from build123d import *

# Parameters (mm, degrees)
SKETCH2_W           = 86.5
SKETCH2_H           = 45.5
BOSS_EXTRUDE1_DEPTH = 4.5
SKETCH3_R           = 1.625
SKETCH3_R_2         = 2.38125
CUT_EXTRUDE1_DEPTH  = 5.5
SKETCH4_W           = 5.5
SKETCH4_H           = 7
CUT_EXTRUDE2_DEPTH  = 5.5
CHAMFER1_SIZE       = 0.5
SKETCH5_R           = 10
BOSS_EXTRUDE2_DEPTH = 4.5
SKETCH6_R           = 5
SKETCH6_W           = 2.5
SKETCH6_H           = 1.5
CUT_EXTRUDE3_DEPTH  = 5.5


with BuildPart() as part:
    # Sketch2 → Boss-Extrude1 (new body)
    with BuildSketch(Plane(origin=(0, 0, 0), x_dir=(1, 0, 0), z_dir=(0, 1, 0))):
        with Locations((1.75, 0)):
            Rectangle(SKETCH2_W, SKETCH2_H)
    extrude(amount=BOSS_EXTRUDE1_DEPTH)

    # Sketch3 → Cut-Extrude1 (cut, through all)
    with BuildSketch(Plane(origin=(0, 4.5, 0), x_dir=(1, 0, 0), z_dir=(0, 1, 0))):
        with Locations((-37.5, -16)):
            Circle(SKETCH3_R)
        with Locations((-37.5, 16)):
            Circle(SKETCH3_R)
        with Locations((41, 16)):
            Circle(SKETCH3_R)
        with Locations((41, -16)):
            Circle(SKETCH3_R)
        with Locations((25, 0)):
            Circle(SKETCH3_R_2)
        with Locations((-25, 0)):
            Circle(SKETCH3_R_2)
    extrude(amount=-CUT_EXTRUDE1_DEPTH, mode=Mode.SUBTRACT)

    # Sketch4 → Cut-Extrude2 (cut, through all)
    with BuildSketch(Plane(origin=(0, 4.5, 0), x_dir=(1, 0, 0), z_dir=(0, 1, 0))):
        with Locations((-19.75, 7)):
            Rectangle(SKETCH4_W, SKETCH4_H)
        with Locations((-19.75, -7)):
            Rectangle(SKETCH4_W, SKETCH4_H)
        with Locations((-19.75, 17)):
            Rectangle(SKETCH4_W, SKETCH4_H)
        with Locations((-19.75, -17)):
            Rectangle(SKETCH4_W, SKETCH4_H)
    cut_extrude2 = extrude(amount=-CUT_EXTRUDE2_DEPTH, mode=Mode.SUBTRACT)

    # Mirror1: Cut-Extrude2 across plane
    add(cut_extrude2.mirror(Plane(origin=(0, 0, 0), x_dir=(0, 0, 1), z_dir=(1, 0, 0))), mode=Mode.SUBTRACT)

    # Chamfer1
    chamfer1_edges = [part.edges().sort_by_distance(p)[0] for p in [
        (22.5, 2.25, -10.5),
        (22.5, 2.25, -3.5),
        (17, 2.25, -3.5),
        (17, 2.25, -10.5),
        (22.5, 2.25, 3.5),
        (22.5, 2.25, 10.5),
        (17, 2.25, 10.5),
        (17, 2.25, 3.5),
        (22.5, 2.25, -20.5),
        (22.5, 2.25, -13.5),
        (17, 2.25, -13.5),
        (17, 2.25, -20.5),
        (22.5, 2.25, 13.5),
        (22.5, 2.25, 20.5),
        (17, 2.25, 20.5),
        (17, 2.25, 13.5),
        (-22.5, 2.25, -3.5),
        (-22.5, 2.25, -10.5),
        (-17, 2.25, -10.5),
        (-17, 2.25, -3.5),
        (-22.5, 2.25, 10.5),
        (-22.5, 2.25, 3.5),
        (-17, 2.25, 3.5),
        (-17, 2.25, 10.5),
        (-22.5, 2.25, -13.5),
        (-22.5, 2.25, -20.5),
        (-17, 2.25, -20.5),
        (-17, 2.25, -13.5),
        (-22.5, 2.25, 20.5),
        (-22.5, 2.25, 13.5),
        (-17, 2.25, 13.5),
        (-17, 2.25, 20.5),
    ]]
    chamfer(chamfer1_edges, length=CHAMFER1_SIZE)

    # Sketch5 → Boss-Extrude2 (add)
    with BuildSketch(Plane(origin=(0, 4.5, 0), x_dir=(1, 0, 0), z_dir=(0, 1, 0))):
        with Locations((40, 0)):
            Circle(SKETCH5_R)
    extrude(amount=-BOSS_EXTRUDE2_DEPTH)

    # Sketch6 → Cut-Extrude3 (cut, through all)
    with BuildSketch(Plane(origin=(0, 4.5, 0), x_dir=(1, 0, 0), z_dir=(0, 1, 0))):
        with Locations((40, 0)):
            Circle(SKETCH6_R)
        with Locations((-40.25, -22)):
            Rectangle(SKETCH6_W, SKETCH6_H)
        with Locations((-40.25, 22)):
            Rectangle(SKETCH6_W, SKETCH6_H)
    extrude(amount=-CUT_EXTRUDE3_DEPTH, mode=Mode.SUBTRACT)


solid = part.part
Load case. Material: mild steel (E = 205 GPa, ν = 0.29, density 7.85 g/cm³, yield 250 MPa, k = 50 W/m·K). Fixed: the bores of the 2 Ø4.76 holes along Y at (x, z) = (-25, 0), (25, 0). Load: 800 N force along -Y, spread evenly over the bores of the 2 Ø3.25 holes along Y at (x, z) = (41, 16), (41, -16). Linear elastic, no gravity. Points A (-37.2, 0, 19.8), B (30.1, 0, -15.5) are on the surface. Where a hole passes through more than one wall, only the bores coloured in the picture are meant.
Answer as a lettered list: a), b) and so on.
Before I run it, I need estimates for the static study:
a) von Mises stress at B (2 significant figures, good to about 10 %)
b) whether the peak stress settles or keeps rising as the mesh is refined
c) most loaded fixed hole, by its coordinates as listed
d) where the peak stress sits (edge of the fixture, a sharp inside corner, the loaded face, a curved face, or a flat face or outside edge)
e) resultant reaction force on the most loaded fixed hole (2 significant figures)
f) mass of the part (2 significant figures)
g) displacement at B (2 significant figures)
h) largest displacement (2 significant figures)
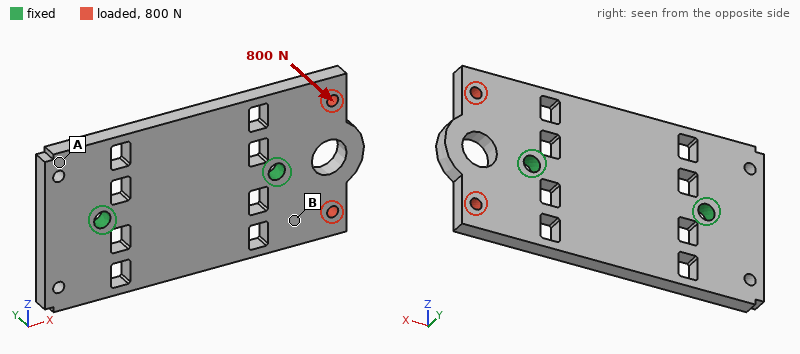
a) 41 MPa
b) keeps rising
c) (25, 0)
d) edge of the fixture
e) 860 N
f) 120 g
g) 18 µm
h) 60 µm
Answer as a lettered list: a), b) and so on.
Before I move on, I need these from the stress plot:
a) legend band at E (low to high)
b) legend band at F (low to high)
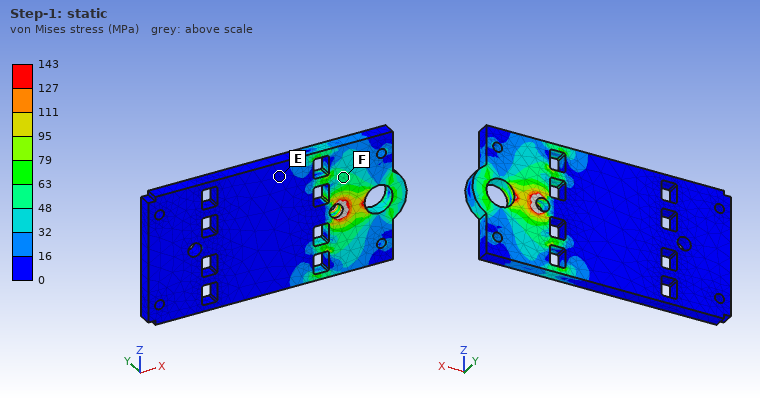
a) 0 to 16 MPa
b) 48 to 63 MPa
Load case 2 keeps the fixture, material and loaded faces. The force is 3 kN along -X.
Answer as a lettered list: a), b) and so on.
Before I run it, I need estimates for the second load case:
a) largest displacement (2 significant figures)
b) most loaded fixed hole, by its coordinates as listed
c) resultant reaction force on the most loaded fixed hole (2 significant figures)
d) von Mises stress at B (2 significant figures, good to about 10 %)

a) 5.8 µm
b) (25, 0)
c) 2.2 kN
d) 15 MPa
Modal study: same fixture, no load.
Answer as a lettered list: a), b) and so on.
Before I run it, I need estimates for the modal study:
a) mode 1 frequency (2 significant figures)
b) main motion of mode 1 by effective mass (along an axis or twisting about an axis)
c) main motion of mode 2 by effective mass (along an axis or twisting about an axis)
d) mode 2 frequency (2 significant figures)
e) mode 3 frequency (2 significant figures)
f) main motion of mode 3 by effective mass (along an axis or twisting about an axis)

a) 4300 Hz
b) twisting about X
c) along Y
d) 5500 Hz
e) 5800 Hz
f) along Y
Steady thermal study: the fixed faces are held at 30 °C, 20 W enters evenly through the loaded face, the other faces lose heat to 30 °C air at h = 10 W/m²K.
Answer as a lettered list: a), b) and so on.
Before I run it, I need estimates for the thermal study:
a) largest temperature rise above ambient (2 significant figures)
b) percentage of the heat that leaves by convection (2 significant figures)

a) 66 K
b) 7.1 %
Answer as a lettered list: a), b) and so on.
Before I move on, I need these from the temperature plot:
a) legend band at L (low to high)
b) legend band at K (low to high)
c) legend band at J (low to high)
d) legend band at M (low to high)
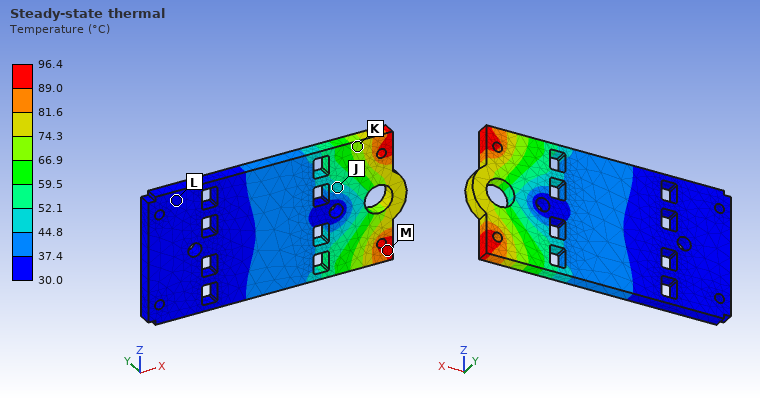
a) 30.0 to 37.4 °C
b) 66.9 to 74.3 °C
c) 44.8 to 52.1 °C
d) 89.0 to 96.4 °C
